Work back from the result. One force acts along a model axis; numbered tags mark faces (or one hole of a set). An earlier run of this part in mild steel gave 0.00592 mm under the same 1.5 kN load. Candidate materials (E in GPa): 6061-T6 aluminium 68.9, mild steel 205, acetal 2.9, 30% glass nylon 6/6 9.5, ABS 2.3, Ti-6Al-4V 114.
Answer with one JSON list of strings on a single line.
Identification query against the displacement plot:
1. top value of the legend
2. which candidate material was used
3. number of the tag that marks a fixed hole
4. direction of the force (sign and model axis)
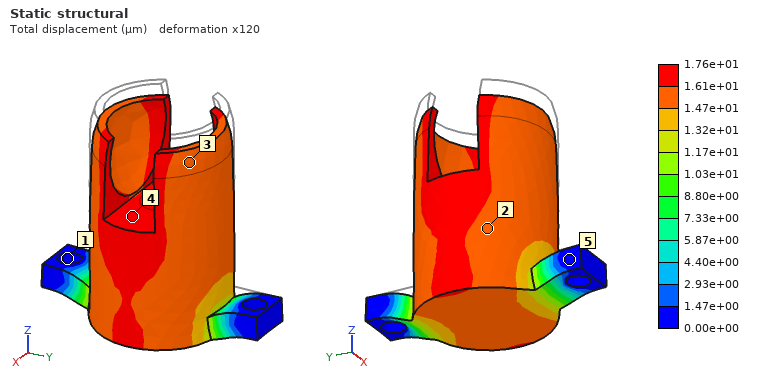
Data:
["1.76e+01 µm", "6061-T6 aluminium", "1", "-Z"]
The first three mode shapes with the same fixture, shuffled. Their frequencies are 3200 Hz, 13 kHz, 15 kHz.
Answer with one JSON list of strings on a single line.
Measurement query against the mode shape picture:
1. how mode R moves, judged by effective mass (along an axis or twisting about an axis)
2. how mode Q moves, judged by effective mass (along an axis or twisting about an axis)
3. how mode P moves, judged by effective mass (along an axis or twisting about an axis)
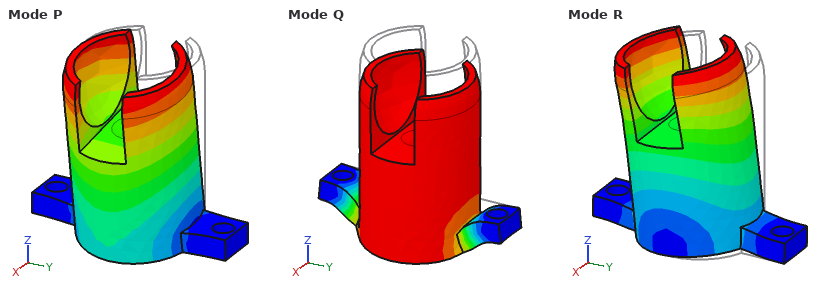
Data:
["along Y", "along Z", "along X"]
